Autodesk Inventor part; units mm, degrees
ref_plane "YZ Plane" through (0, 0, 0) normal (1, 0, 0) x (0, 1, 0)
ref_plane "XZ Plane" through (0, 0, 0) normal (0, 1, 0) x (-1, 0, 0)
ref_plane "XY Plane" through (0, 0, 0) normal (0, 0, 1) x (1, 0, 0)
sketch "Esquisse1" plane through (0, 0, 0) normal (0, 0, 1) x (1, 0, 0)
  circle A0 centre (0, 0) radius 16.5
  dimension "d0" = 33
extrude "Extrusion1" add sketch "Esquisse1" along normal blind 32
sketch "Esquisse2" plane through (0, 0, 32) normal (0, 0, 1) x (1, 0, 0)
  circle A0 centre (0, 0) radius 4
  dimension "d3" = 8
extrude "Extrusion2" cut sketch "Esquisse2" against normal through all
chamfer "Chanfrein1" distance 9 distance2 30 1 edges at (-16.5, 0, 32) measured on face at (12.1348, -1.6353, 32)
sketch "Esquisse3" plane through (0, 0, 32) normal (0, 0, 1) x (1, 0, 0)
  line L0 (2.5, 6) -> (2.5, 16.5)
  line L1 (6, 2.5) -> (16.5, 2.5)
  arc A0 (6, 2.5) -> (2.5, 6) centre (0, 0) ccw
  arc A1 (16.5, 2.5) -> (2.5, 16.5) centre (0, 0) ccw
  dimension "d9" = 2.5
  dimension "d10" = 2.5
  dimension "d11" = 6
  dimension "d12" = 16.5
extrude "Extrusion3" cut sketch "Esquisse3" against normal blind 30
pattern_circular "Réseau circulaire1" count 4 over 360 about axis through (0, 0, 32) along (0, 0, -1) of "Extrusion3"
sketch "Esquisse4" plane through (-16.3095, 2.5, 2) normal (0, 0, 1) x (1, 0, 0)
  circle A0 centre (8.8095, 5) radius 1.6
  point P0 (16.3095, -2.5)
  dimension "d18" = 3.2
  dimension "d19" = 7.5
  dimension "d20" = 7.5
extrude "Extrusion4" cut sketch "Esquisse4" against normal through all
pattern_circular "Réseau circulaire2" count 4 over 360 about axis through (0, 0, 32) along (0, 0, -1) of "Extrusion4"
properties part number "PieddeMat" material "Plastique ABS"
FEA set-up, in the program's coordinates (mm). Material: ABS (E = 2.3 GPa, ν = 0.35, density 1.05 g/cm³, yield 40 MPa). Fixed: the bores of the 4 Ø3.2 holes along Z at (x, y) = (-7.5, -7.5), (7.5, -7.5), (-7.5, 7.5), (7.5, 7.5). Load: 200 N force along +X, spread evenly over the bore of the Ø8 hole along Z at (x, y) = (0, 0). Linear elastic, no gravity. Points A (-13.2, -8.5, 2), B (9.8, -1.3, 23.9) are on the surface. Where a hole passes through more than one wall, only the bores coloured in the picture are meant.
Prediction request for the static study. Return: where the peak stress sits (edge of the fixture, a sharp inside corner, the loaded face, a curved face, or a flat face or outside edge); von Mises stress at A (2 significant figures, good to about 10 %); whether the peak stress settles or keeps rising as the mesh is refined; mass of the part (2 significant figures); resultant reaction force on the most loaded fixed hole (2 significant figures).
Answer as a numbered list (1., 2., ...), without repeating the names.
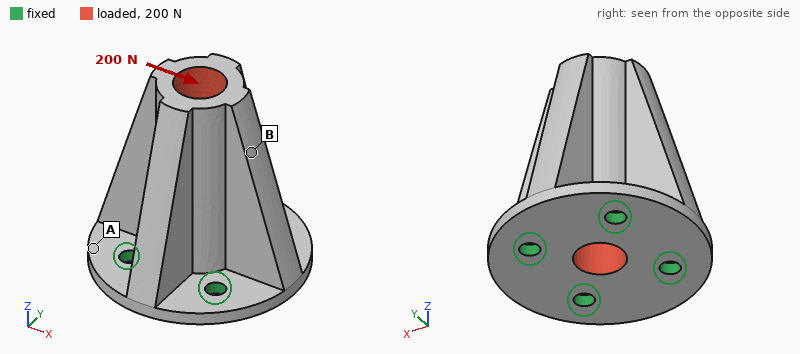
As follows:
1. edge of the fixture
2. 6.4 MPa
3. keeps rising
4. 7.7 g
5. 110 N
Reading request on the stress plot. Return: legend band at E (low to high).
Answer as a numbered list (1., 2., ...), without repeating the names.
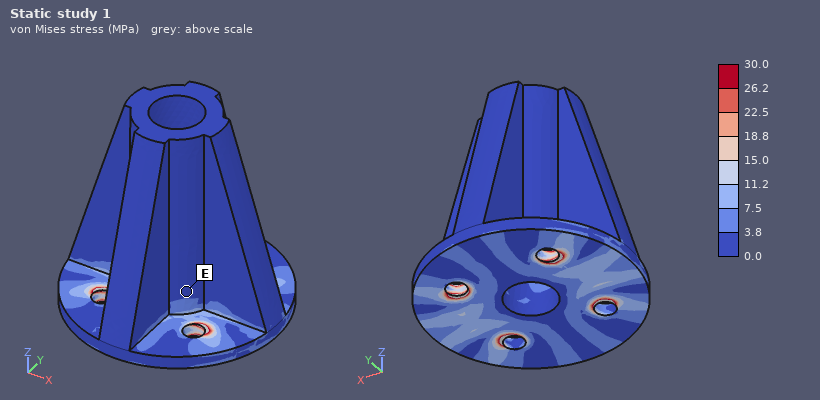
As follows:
1. 0.0 to 3.8 MPa
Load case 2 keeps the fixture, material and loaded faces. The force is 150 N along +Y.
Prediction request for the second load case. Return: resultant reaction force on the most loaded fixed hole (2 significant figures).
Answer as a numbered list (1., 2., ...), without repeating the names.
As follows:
1. 85 N
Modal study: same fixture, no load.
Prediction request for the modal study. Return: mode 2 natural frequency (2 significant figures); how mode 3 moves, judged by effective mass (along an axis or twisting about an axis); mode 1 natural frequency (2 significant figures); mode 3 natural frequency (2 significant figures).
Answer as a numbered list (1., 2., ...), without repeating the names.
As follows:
1. 2100 Hz
2. along Z
3. 2100 Hz
4. 5200 Hz
